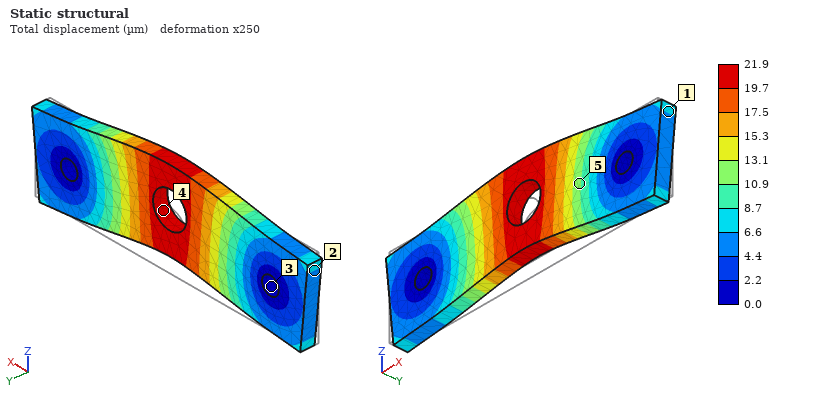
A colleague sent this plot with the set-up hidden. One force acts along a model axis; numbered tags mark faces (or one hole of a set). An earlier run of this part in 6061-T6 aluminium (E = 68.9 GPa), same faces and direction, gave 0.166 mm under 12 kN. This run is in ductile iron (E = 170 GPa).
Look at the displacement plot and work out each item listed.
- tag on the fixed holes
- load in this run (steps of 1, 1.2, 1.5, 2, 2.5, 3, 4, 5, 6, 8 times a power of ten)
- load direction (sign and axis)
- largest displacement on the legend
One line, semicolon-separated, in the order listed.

3; 4 kN; +Z; 21.9 µm
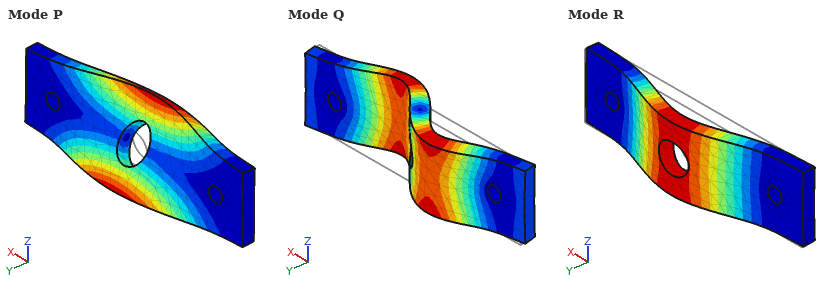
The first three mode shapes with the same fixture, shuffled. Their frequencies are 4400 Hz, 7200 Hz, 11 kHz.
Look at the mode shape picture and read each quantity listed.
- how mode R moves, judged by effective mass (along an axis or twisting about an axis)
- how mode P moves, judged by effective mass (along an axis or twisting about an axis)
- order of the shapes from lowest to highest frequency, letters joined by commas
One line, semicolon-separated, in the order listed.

along Y; twisting about X; R, P, Q
